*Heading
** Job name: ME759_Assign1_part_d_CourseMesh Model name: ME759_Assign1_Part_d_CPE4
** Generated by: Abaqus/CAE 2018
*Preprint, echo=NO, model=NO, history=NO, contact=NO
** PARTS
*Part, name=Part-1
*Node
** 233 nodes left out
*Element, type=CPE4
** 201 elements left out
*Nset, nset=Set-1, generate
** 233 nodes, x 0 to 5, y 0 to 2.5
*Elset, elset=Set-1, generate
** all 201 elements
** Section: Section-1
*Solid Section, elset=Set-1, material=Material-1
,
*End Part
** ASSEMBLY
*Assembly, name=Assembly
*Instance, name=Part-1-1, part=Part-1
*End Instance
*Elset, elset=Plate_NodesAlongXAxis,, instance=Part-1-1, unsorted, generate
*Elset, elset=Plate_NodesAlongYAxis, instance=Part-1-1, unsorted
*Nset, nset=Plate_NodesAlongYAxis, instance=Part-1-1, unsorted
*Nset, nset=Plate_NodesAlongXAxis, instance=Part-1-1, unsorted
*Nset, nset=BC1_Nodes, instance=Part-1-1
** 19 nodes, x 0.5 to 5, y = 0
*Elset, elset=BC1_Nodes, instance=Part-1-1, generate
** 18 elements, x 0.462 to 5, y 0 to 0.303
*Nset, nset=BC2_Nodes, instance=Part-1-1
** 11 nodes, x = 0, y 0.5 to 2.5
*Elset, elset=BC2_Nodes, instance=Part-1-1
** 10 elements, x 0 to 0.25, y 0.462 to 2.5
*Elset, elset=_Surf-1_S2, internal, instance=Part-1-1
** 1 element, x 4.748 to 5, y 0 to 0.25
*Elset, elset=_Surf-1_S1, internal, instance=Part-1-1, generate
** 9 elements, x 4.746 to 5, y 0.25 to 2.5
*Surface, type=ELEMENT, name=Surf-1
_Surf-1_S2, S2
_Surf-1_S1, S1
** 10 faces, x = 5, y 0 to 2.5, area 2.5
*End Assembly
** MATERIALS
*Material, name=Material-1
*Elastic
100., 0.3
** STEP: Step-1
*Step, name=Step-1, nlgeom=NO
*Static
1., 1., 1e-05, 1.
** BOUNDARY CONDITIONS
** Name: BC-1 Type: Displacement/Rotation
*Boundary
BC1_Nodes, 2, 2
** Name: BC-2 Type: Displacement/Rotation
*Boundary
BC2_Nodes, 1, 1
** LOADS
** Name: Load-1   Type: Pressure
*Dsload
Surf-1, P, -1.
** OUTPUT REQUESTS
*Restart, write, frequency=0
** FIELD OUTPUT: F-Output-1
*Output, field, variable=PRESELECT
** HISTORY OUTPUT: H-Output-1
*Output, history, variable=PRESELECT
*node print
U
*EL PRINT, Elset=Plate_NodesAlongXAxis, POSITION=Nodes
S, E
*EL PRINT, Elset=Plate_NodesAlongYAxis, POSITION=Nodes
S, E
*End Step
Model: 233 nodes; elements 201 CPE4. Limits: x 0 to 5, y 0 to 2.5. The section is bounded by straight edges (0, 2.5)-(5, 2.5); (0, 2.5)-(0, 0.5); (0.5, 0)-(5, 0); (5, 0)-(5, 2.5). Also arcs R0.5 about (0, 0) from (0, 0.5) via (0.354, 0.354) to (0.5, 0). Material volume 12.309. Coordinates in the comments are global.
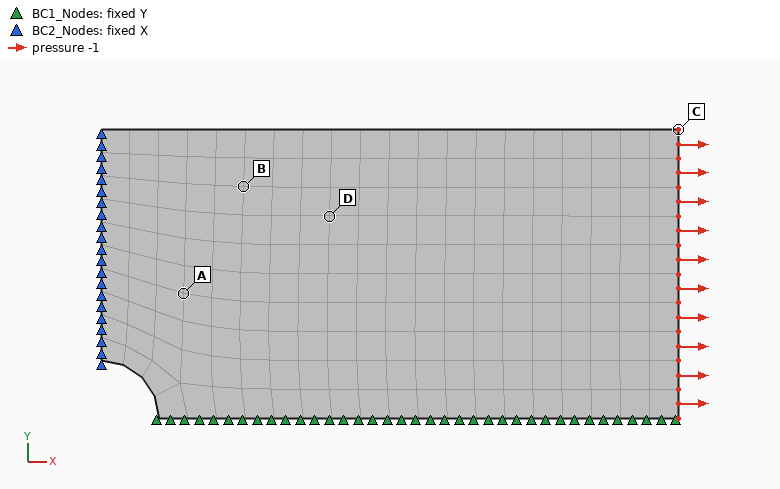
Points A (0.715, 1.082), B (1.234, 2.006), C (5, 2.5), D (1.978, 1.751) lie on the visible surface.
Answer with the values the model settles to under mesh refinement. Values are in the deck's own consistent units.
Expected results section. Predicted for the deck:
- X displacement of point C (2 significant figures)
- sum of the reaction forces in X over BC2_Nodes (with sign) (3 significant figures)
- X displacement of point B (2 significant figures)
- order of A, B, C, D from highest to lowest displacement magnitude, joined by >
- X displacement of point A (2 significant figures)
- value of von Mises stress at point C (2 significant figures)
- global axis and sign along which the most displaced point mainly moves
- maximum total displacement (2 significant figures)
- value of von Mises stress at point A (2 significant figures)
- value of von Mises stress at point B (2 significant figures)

0.047
-2.50
0.012
C > D > B > A
0.0077
0.89
+X
0.048
1.1
0.98
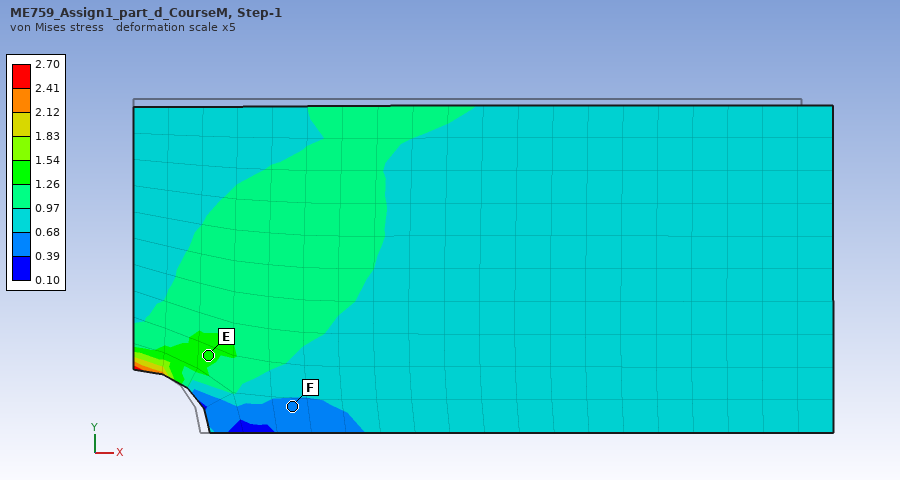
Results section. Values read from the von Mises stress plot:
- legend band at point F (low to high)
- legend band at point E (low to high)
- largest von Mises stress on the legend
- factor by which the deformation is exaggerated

0.39 to 0.68
1.26 to 1.54
2.70
5
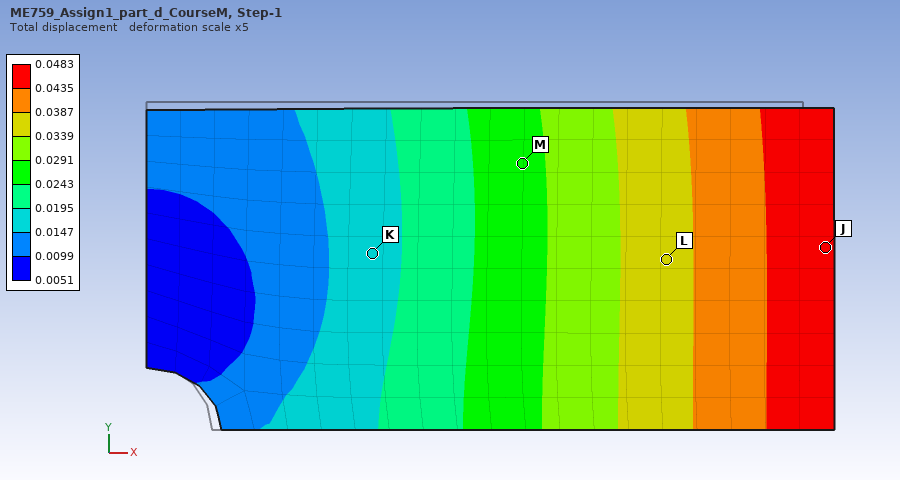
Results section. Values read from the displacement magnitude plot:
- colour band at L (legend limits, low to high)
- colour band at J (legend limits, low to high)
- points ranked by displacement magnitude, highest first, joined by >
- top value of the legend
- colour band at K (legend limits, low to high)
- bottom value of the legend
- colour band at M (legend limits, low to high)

0.0339 to 0.0387
0.0435 to 0.0483
J > L > M > K
0.0483
0.0147 to 0.0195
0.0051
0.0243 to 0.0291
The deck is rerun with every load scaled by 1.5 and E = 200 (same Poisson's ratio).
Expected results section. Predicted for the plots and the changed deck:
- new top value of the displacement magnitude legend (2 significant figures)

0.036
